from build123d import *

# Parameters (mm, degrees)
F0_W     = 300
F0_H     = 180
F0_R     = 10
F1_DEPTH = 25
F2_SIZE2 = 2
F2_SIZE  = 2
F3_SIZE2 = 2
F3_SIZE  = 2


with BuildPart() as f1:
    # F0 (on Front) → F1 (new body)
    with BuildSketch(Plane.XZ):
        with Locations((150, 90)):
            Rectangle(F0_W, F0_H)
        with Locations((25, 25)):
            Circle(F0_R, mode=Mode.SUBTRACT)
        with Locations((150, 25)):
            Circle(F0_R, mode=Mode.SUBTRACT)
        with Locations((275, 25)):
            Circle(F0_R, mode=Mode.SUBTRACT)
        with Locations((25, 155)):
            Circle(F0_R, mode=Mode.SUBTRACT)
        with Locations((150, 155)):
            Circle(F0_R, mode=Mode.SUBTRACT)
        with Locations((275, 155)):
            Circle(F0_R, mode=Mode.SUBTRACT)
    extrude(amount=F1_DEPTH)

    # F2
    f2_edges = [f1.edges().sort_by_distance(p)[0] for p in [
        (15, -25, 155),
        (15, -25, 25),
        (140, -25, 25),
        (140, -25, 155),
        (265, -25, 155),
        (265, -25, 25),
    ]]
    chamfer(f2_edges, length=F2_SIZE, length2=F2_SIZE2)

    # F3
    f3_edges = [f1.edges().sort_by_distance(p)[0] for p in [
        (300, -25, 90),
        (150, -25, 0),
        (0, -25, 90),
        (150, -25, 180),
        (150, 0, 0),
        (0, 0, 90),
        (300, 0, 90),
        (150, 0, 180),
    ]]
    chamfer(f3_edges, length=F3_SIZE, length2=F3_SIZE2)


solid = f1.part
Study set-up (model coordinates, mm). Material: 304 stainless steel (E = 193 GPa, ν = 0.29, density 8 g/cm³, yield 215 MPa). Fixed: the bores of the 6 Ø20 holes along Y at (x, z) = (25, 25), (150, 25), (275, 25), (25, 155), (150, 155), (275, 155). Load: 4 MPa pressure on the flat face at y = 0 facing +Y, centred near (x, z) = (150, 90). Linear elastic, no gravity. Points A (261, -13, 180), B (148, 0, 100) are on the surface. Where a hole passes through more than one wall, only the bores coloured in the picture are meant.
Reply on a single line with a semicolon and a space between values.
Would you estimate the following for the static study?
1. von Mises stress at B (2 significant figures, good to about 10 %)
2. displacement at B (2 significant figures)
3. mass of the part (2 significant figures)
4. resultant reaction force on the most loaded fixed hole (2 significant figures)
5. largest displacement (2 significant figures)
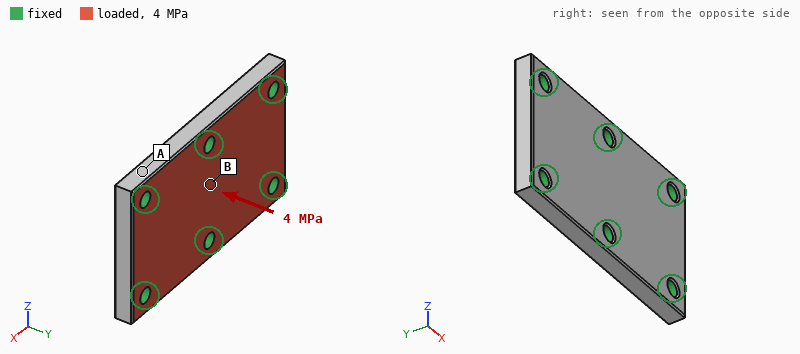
32 MPa; 23 µm; 10 kg; 44 kN; 29 µm
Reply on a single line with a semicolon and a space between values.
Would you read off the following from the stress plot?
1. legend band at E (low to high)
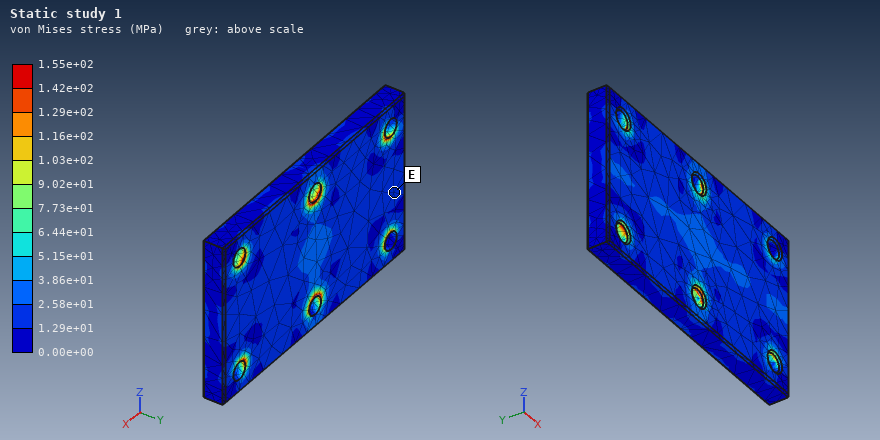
1.29e+01 to 2.58e+01 MPa
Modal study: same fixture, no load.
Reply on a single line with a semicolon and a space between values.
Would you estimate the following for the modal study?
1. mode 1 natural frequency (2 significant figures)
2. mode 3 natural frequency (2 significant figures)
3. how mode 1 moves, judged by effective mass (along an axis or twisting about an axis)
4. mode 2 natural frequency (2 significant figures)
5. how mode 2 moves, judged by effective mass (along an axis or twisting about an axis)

5000 Hz; 7400 Hz; along Y; 5200 Hz; twisting about Z
